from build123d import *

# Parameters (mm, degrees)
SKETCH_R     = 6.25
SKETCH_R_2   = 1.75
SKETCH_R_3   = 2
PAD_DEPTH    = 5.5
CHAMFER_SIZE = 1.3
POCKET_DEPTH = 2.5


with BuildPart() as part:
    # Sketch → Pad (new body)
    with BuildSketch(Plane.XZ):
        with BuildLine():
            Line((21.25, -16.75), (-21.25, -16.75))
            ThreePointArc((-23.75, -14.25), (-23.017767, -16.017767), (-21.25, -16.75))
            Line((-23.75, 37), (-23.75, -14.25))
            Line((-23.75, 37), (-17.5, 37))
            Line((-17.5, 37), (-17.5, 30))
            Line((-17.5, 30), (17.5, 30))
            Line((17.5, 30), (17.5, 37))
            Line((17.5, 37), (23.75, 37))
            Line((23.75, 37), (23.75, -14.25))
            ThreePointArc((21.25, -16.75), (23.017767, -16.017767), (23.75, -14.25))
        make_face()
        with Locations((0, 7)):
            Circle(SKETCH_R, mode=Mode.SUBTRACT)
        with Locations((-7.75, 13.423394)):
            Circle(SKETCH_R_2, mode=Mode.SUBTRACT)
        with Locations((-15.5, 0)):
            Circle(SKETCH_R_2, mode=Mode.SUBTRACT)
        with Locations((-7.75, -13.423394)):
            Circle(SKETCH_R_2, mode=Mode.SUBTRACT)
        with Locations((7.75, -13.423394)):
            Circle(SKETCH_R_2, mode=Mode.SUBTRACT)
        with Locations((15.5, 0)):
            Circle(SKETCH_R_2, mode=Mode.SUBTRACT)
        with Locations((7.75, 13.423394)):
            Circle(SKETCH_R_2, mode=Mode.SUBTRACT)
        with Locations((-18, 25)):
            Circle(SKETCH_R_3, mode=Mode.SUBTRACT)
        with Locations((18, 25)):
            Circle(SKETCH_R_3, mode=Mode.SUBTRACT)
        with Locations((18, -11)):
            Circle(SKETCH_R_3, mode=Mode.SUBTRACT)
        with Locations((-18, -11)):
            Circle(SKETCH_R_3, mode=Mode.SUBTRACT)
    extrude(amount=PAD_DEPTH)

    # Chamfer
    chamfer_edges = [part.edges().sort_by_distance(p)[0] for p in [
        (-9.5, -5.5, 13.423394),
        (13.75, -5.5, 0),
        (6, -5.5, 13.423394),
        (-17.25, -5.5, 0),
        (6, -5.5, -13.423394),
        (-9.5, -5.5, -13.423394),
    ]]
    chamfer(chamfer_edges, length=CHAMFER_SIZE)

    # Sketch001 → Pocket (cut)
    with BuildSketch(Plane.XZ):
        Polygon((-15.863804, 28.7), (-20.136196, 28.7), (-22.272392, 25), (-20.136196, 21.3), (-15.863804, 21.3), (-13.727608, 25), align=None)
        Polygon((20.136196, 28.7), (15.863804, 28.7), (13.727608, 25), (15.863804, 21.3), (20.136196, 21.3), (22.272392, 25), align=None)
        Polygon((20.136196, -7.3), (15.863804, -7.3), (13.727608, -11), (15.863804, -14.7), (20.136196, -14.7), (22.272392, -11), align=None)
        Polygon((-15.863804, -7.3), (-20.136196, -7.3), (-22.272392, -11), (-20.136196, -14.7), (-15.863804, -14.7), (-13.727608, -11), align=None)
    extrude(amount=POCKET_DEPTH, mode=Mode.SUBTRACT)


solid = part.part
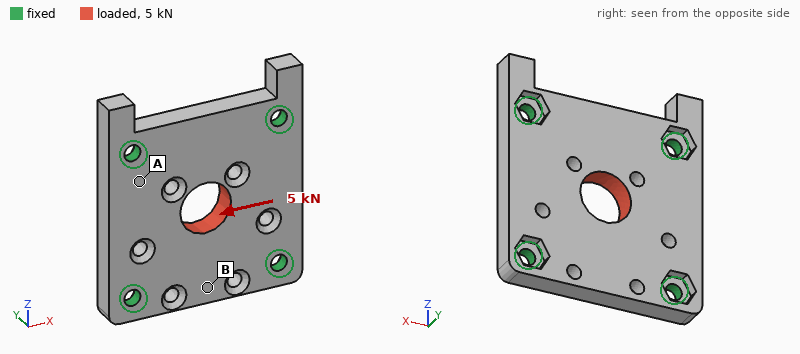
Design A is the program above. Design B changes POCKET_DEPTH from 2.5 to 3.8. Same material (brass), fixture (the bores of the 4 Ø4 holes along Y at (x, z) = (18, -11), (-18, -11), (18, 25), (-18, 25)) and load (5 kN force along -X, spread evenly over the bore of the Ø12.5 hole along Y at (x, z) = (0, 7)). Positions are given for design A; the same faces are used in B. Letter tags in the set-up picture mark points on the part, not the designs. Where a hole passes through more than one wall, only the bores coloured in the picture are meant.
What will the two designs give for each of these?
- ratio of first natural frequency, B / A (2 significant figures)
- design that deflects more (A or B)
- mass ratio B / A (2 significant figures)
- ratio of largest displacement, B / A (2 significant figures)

0.90
B
0.98
1.2
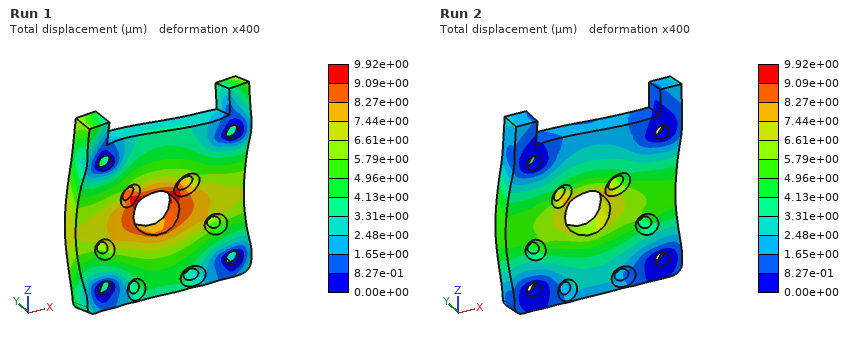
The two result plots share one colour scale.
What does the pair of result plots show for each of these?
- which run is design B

Run 1
